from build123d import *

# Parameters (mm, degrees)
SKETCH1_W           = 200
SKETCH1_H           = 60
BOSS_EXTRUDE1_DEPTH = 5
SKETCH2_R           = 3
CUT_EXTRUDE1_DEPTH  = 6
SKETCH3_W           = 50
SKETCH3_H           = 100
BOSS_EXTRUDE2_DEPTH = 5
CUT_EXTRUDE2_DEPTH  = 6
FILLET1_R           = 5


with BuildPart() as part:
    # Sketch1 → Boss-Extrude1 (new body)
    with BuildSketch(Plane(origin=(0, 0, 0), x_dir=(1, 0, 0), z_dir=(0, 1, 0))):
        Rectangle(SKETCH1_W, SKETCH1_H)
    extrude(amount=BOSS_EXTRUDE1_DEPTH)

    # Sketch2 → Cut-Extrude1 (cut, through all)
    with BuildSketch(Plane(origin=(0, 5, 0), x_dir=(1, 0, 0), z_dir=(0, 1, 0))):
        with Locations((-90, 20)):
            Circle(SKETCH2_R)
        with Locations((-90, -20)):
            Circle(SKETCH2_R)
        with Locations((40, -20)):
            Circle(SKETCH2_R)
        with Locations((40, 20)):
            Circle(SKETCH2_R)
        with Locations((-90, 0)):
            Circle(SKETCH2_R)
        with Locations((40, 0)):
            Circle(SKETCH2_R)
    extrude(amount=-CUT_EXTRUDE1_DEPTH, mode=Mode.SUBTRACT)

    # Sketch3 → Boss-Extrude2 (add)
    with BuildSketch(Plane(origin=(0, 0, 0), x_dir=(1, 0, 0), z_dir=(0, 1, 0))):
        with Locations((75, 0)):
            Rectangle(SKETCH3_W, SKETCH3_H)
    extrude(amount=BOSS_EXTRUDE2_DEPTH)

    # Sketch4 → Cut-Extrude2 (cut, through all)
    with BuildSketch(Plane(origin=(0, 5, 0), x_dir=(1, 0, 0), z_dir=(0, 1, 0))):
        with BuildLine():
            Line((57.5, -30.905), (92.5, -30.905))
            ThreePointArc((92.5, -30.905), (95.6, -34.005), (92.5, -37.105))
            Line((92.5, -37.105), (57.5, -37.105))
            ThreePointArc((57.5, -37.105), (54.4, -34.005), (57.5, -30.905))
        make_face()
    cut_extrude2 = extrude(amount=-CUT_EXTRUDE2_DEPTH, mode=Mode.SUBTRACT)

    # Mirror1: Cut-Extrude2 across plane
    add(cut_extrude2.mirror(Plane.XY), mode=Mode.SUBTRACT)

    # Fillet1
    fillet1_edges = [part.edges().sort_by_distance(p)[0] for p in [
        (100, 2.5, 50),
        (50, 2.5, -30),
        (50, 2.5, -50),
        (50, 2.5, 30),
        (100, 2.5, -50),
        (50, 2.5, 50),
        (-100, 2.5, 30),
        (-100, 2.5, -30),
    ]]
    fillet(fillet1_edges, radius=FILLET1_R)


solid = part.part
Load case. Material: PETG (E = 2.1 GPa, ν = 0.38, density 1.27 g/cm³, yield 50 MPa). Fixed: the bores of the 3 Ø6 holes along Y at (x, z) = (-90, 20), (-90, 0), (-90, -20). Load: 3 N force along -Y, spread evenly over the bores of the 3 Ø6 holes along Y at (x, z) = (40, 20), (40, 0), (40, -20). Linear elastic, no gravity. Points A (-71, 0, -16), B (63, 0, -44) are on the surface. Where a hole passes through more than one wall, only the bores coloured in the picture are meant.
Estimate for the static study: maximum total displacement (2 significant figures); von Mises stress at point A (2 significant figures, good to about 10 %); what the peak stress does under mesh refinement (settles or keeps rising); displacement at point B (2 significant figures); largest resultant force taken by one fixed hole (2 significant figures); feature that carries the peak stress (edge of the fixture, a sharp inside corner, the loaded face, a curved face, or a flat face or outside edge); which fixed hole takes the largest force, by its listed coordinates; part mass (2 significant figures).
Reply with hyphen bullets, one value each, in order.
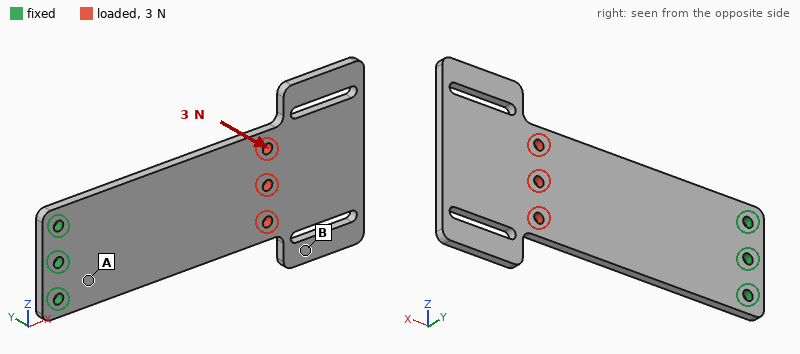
- 2.7 mm
- 1.2 MPa
- keeps rising
- 2.0 mm
- 4.3 N
- edge of the fixture
- (-90, 0)
- 85 g
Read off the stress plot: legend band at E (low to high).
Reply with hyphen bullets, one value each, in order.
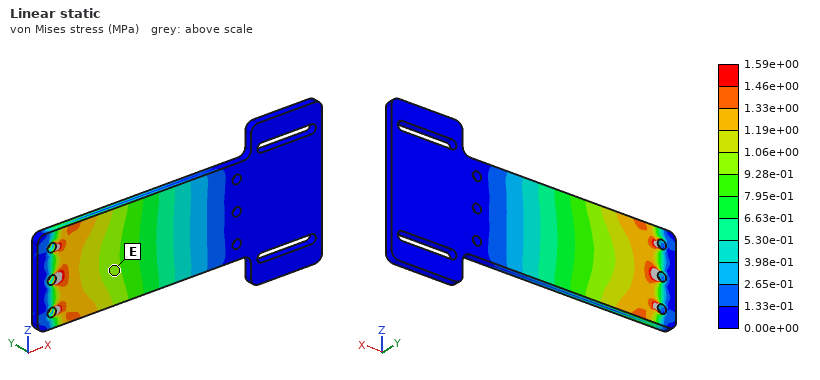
- 9.28e-01 to 1.06e+00 MPa
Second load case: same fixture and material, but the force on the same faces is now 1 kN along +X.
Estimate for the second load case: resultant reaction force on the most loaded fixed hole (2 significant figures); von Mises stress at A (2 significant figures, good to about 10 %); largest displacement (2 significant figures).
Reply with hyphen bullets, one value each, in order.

- 350 N
- 3.4 MPa
- 0.22 mm
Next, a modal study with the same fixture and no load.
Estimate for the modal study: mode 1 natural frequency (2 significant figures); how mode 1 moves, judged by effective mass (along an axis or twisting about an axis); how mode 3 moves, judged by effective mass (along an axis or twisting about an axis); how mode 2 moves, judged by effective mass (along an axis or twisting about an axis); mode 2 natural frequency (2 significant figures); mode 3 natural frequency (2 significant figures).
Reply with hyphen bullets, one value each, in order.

- 26 Hz
- along Y
- along Y
- twisting about X
- 110 Hz
- 170 Hz
